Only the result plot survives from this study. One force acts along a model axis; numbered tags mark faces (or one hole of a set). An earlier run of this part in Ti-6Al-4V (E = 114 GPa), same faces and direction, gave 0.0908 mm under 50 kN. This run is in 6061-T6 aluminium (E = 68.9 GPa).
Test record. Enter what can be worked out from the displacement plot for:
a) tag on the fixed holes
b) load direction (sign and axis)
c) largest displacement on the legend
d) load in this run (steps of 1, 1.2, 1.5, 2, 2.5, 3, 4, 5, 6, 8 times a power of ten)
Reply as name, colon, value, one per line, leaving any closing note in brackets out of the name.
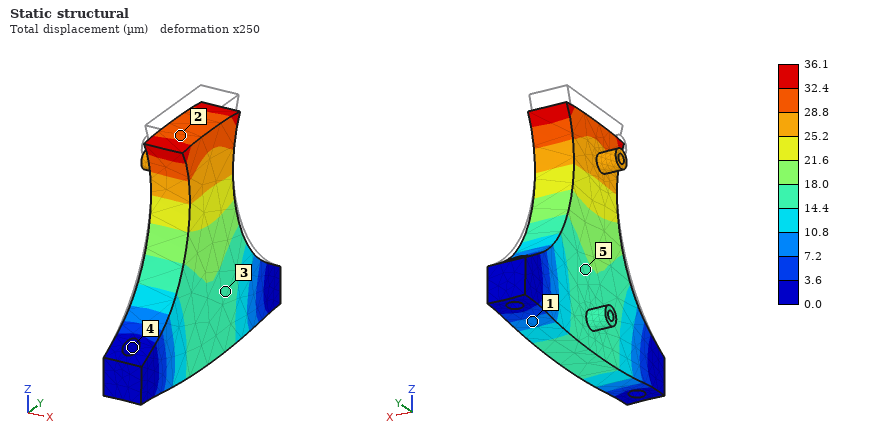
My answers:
tag on the fixed holes: 4
load direction: -Z
largest displacement on the legend: 36.1 µm
load in this run: 12 kN
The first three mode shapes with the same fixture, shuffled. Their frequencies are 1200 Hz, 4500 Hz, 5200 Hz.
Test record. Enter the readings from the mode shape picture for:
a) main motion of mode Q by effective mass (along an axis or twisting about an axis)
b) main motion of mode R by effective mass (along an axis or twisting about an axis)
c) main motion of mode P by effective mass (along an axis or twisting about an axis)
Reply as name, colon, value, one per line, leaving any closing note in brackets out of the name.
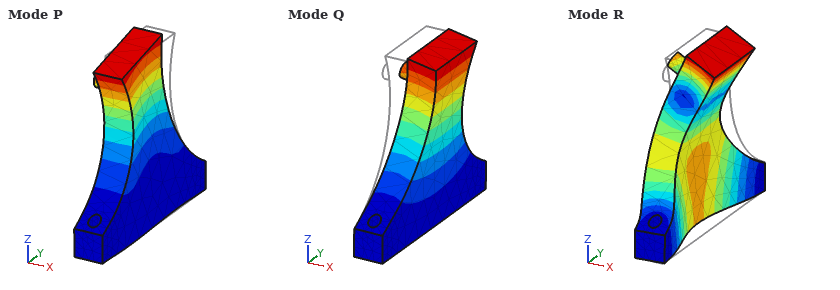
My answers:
main motion of mode Q by effective mass: along X
main motion of mode R by effective mass: along X
main motion of mode P by effective mass: along Y
